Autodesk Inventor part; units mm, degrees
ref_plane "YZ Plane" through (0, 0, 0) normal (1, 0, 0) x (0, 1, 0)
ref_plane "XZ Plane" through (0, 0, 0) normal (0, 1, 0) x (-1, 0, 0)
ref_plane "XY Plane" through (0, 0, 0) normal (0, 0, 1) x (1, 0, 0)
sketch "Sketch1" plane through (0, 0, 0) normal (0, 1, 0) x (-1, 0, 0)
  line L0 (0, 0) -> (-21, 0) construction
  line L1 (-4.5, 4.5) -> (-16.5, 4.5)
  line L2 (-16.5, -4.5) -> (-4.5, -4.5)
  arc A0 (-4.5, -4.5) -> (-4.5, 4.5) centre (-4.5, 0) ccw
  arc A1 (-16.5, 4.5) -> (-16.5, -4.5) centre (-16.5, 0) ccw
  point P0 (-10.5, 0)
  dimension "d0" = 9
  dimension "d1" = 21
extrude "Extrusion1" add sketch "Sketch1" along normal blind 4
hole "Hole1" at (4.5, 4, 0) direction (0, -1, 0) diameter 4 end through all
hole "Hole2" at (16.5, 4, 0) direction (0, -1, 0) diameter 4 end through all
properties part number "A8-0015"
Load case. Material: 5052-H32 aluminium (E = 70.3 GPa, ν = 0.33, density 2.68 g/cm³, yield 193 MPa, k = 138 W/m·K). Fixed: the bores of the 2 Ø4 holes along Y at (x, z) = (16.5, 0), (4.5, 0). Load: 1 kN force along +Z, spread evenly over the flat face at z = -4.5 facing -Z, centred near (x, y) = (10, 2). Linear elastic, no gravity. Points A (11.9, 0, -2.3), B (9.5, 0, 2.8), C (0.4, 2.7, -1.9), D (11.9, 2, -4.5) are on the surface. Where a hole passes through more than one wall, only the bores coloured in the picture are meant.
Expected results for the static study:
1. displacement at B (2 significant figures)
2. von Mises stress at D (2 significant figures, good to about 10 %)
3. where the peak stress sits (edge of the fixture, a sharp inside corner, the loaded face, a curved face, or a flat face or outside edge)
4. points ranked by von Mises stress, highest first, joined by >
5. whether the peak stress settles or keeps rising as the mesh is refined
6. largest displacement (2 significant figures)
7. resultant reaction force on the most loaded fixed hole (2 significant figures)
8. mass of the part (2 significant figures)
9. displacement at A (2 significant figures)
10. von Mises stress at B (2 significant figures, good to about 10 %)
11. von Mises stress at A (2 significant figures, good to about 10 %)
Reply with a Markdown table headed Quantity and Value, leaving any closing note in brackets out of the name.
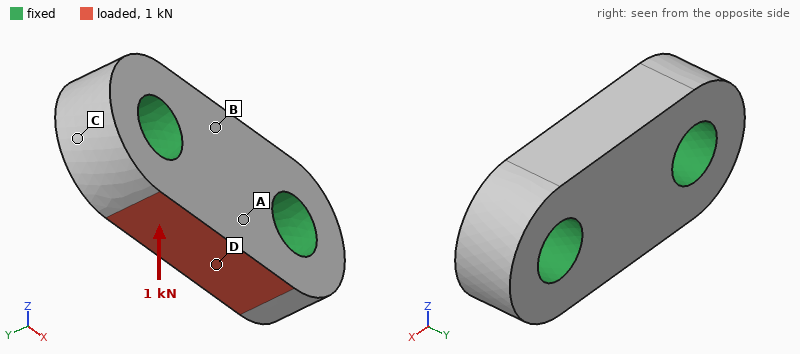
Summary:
| Quantity | Value |
|---|---|
| displacement at B | 0.99 µm |
| von Mises stress at D | 21 MPa |
| where the peak stress sits | edge of the fixture |
| points ranked by von Mises stress, highest first, joined by > | D > A > B > C |
| whether the peak stress settles or keeps rising as the mesh is refined | keeps rising |
| largest displacement | 2.2 µm |
| resultant reaction force on the most loaded fixed hole | 520 N |
| mass of the part | 1.6 g |
| displacement at A | 1.6 µm |
| von Mises stress at B | 7.3 MPa |
| von Mises stress at A | 16 MPa |
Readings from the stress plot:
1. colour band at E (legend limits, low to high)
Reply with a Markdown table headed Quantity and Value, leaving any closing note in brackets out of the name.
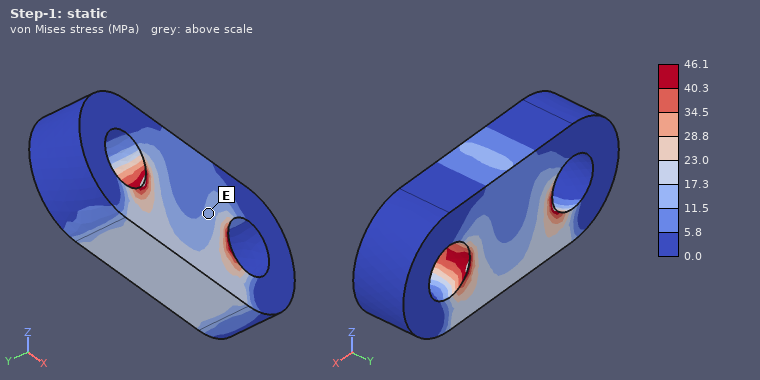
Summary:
| Quantity | Value |
|---|---|
| colour band at E | 11.5 to 17.3 MPa |
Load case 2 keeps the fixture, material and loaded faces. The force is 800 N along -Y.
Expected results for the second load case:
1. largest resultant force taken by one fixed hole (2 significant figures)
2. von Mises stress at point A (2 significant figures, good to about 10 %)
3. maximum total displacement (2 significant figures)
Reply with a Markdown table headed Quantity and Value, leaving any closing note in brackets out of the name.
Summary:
| Quantity | Value |
|---|---|
| largest resultant force taken by one fixed hole | 400 N |
| von Mises stress at point A | 39 MPa |
| maximum total displacement | 9.0 µm |
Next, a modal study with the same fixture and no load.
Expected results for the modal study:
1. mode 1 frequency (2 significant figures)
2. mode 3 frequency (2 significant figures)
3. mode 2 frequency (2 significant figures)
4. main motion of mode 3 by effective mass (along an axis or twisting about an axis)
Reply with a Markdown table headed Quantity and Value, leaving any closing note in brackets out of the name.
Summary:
| Quantity | Value |
|---|---|
| mode 1 frequency | 120 kHz |
| mode 3 frequency | 140 kHz |
| mode 2 frequency | 120 kHz |
| main motion of mode 3 by effective mass | along Z |
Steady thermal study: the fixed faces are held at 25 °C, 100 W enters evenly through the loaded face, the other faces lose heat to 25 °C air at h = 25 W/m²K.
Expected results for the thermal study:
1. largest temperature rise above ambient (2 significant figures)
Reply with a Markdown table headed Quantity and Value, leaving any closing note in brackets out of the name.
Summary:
| Quantity | Value |
|---|---|
| largest temperature rise above ambient | 64 K |
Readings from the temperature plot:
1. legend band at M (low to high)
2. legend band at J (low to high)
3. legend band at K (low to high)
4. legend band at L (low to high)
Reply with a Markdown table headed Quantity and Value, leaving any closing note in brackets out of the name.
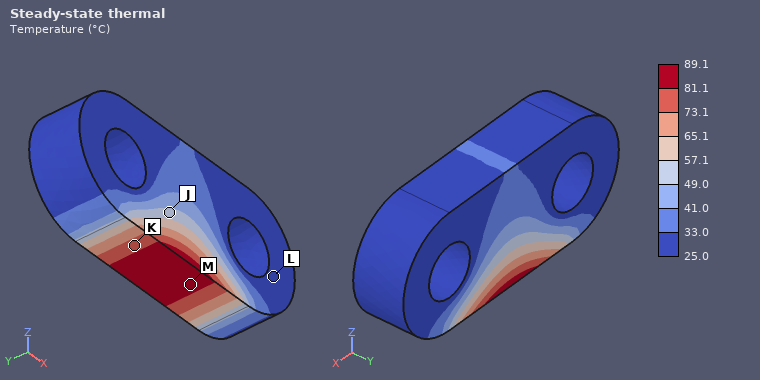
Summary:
| Quantity | Value |
|---|---|
| legend band at M | 81.1 to 89.1 °C |
| legend band at J | 49.0 to 57.1 °C |
| legend band at K | 73.1 to 81.1 °C |
| legend band at L | 25.0 to 33.0 °C |
